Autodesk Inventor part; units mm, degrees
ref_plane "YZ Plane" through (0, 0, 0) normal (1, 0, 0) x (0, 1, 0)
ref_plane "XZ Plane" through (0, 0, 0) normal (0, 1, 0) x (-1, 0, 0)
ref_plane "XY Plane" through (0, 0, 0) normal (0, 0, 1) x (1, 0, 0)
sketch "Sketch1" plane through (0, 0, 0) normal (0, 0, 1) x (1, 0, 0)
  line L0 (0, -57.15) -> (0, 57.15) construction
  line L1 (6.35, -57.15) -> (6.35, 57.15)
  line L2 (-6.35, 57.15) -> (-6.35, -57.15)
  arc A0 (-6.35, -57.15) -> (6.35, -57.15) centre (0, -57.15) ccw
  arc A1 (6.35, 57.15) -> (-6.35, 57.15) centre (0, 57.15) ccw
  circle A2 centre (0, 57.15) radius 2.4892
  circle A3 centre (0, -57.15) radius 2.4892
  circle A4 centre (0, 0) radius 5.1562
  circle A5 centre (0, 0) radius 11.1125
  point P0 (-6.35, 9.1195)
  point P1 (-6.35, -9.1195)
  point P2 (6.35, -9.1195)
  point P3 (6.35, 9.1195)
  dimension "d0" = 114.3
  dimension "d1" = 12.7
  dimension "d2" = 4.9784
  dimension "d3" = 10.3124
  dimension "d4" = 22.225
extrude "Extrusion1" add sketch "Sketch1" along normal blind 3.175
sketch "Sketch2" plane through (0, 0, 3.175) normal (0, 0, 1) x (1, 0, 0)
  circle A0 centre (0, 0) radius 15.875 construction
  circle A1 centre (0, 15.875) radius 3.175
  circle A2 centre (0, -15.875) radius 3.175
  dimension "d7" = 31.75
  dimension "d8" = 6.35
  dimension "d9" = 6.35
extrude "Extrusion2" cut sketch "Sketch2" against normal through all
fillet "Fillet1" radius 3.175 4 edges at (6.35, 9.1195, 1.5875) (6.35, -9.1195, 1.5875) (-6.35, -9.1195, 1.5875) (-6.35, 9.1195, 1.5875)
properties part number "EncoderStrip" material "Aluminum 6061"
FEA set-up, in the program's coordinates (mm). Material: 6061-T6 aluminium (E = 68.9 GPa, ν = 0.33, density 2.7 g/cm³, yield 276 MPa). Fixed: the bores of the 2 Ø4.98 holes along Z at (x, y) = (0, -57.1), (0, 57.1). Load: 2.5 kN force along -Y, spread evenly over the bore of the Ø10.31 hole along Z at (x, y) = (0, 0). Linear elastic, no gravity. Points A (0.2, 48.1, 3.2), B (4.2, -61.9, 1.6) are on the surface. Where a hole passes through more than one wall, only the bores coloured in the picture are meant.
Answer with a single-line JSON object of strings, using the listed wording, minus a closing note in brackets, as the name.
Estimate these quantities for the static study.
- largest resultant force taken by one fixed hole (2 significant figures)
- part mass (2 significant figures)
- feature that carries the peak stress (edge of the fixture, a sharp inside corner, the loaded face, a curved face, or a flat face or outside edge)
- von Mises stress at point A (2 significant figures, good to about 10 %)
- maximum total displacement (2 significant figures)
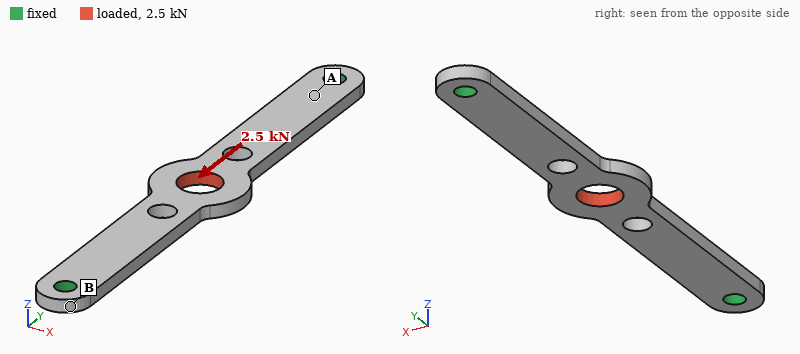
{"largest resultant force taken by one fixed hole": "1.3 kN", "part mass": "13 g", "feature that carries the peak stress": "a curved face", "von Mises stress at point A": "35 MPa", "maximum total displacement": "30 µm"}
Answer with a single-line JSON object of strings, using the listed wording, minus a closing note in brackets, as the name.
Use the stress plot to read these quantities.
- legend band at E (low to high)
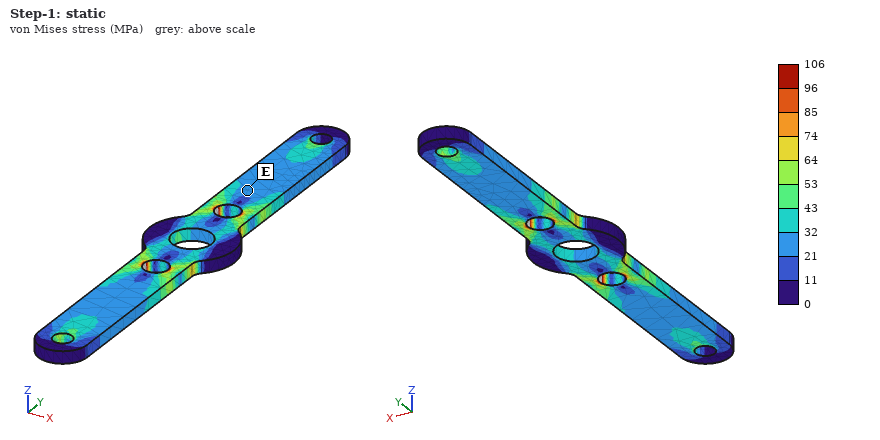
{"legend band at E": "21 to 32 MPa"}
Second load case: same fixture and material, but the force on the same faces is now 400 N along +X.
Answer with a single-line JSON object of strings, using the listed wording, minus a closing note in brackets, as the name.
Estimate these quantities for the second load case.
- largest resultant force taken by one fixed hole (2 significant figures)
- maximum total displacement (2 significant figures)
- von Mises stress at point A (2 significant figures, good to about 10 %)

{"largest resultant force taken by one fixed hole": "200 N", "maximum total displacement": "96 µm", "von Mises stress at point A": "13 MPa"}
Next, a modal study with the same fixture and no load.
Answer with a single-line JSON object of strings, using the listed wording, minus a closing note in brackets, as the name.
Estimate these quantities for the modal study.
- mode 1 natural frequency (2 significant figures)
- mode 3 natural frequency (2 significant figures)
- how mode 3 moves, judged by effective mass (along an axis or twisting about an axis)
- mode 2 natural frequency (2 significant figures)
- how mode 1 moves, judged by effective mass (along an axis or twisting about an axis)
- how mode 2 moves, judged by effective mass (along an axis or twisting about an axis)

{"mode 1 natural frequency": "1300 Hz", "mode 3 natural frequency": "4500 Hz", "how mode 3 moves, judged by effective mass": "along X", "mode 2 natural frequency": "3500 Hz", "how mode 1 moves, judged by effective mass": "along Z", "how mode 2 moves, judged by effective mass": "twisting about X"}
